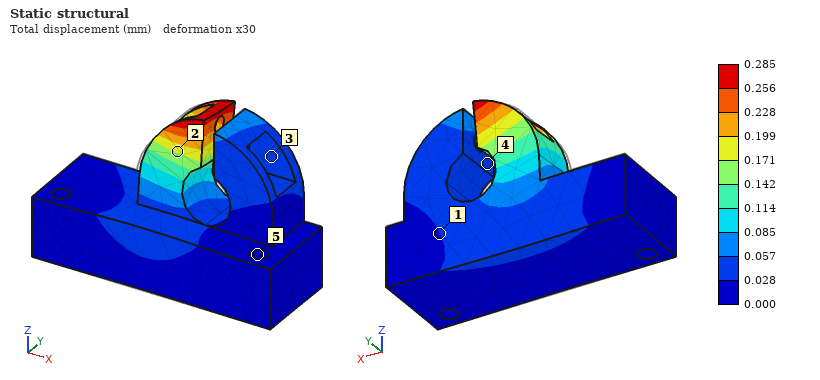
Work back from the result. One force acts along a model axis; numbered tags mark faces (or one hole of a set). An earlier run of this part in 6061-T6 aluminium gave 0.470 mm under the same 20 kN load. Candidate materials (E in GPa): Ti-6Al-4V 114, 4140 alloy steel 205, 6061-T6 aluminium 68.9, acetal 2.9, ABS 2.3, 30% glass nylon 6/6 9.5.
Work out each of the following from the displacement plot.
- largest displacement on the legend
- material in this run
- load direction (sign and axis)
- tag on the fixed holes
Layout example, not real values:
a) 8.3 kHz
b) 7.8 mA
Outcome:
a) 0.285 mm
b) Ti-6Al-4V
c) +Y
d) 5
